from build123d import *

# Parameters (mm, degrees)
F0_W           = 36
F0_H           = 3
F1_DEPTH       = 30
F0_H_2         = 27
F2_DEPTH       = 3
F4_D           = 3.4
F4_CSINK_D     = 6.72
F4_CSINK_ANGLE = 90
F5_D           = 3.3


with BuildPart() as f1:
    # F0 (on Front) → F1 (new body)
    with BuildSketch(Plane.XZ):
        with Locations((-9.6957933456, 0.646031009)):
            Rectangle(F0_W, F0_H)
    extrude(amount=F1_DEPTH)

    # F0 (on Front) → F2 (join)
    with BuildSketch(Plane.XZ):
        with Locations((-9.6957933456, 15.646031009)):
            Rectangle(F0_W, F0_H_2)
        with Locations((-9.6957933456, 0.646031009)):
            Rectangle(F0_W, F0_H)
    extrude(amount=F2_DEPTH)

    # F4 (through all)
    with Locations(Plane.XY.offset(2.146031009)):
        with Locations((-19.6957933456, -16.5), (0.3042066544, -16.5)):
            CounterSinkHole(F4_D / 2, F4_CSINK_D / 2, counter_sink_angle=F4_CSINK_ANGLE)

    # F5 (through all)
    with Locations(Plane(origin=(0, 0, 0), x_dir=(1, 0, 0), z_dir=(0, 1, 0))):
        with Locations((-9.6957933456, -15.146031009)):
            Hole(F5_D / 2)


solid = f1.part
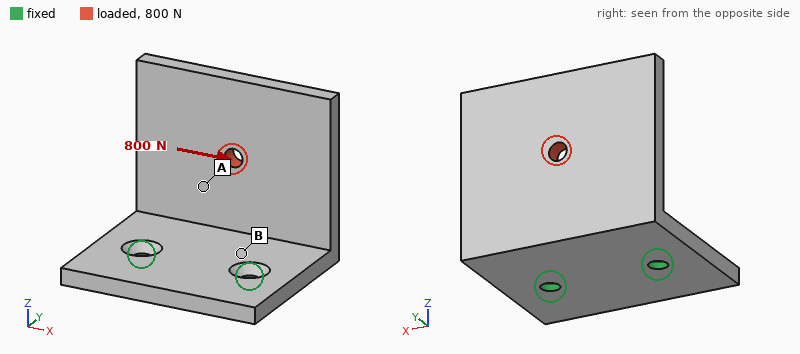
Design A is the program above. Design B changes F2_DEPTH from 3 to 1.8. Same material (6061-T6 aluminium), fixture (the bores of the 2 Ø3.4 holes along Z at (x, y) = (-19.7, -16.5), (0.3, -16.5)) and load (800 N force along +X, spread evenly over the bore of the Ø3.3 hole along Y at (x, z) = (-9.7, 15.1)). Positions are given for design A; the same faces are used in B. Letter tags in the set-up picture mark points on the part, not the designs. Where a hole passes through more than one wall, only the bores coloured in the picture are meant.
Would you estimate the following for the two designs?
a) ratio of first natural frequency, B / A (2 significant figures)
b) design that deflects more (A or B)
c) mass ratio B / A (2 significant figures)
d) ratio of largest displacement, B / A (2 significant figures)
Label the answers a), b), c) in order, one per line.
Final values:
a) 1.0
b) B
c) 0.81
d) 1.4
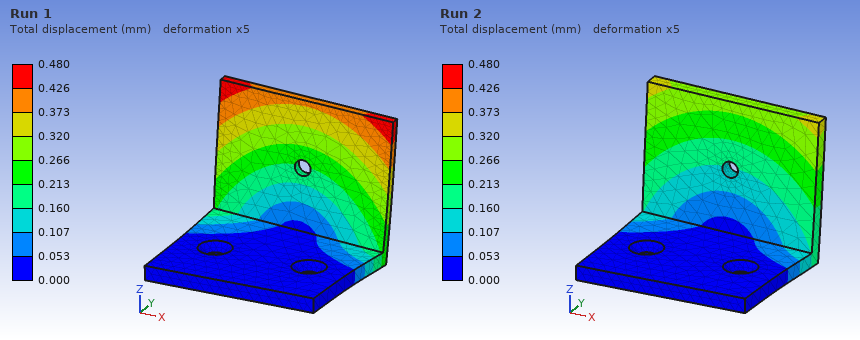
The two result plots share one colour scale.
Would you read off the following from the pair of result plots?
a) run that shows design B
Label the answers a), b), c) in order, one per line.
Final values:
a) Run 1
